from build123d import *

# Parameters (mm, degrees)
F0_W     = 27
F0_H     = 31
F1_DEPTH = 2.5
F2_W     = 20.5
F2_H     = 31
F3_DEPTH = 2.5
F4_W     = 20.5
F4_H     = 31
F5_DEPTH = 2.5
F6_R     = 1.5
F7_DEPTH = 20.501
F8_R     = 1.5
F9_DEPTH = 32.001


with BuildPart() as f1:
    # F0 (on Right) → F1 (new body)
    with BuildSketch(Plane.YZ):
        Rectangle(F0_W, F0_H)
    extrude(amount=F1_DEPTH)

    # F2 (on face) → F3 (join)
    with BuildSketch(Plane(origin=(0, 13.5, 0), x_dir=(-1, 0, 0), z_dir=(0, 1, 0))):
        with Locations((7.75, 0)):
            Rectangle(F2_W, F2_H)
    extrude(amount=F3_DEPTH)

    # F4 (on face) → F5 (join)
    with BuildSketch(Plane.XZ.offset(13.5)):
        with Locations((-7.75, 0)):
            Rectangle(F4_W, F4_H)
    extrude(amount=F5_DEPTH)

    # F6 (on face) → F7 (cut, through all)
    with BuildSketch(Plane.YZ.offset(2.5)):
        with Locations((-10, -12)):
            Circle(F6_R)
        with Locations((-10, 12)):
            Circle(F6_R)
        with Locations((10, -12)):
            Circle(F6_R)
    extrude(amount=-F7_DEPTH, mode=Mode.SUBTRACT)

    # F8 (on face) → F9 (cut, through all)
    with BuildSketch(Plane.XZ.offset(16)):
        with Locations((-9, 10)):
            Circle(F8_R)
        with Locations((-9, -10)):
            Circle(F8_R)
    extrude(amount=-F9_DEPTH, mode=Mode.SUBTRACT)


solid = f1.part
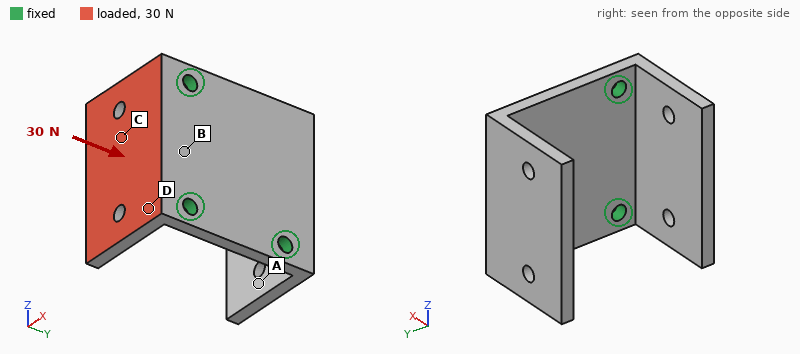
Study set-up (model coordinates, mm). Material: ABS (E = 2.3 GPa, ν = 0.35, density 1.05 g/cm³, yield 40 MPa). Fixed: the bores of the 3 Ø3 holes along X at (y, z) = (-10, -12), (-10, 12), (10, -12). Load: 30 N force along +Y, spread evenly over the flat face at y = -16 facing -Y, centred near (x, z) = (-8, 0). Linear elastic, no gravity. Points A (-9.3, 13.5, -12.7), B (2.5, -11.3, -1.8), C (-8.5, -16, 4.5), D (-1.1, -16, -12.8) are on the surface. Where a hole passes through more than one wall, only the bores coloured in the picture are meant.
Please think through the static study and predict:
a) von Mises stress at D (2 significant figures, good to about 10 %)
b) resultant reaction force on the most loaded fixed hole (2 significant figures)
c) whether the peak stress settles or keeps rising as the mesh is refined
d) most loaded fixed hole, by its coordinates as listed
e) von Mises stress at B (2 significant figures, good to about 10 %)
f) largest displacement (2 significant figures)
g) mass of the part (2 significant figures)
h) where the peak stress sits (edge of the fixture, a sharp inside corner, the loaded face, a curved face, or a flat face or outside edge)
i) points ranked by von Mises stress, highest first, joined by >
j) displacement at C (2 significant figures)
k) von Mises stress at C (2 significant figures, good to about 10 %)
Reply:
5.8 MPa
14 N
keeps rising
(-10, 12)
4.7 MPa
0.48 mm
5.4 g
edge of the fixture
D > B > C > A
0.22 mm
2.0 MPa
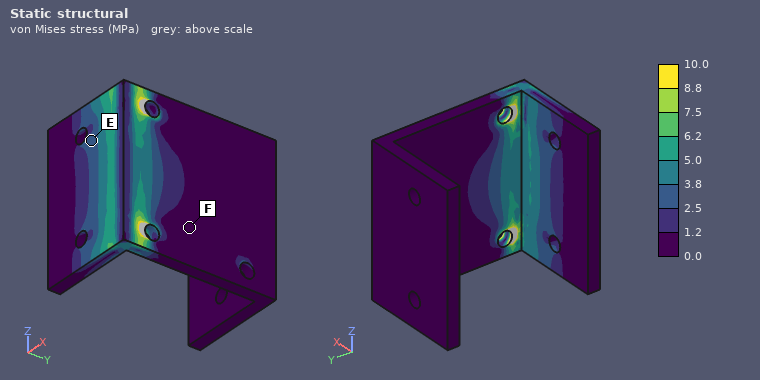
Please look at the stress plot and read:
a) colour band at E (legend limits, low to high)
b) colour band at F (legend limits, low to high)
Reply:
2.5 to 3.8 MPa
0.0 to 1.2 MPa
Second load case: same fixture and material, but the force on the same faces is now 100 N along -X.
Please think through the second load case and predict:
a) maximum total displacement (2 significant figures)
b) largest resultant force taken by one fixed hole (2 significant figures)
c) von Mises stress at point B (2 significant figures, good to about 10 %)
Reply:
0.49 mm
54 N
5.0 MPa
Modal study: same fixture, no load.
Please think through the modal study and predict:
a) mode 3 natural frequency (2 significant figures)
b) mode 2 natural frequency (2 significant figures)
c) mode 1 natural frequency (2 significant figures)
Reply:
1300 Hz
1200 Hz
840 Hz
